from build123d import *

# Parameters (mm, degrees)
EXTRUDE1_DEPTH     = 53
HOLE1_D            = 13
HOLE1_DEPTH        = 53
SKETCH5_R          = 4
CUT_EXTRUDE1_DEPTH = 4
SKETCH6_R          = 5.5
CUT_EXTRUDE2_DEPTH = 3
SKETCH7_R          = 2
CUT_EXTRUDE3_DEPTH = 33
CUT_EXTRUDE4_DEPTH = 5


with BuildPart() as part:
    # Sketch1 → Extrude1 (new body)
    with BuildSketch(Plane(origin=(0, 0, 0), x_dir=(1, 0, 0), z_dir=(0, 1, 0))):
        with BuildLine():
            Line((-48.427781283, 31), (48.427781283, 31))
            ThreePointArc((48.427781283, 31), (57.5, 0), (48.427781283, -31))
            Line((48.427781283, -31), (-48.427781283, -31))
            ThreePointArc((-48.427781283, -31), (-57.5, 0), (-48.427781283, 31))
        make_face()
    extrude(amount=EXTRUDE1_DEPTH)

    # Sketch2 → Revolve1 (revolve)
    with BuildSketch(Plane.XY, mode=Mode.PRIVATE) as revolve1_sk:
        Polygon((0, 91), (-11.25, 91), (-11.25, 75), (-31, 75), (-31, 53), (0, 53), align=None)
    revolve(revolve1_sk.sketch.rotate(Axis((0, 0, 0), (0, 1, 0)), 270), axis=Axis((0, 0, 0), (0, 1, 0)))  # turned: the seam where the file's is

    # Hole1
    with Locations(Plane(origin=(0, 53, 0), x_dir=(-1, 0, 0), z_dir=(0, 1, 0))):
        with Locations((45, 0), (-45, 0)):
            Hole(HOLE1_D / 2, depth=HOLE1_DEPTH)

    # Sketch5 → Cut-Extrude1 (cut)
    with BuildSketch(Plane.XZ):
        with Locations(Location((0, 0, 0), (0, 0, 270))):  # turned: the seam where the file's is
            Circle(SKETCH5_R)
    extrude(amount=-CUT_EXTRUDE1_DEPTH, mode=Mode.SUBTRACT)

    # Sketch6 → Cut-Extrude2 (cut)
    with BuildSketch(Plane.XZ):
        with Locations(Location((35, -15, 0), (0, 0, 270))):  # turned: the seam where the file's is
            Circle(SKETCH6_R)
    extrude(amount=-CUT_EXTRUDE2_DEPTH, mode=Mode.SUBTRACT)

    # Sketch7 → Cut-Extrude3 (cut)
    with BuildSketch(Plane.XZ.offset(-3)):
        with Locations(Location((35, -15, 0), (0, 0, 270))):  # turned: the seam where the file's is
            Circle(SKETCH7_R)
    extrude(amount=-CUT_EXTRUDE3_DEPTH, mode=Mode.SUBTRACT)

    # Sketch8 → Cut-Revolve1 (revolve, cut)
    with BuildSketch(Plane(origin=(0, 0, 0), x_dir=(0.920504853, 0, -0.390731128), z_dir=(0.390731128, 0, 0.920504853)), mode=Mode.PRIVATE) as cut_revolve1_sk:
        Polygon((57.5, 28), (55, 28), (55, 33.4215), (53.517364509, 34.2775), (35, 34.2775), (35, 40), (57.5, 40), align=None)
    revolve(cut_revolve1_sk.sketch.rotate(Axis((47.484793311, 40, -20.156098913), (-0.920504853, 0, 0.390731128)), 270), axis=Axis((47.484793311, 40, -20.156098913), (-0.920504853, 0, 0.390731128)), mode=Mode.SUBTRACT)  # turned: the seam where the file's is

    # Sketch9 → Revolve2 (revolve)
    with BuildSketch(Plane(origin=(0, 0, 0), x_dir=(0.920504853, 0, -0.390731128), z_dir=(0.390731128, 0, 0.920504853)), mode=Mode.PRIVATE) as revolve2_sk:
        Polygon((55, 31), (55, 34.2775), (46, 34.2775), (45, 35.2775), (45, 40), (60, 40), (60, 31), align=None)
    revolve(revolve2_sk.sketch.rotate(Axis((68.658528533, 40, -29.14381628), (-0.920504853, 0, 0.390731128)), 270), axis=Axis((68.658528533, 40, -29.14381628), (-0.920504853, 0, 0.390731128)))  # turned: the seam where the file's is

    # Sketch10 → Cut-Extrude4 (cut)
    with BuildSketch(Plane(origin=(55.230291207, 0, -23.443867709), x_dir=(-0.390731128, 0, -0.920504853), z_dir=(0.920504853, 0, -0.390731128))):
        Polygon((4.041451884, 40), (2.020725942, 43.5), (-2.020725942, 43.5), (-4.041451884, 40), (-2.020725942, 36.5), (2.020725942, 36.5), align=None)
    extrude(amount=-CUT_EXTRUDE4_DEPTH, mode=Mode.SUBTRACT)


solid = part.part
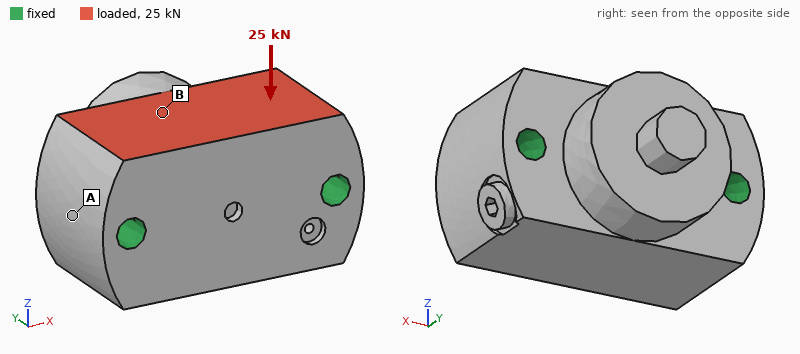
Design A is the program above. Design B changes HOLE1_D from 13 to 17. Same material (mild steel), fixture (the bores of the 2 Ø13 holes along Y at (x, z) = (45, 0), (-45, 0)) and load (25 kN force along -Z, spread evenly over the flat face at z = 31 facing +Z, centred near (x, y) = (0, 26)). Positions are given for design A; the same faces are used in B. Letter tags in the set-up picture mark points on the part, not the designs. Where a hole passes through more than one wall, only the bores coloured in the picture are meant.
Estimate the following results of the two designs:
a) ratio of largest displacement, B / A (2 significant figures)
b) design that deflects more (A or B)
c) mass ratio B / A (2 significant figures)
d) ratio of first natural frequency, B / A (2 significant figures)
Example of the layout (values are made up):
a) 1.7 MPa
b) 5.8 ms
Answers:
a) 0.90
b) A
c) 0.98
d) 1.1
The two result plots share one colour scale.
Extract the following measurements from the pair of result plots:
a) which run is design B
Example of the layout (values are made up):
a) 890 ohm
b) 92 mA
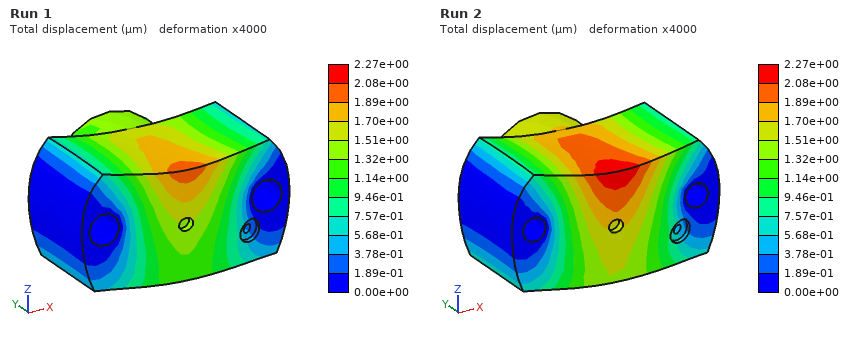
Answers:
a) Run 1
